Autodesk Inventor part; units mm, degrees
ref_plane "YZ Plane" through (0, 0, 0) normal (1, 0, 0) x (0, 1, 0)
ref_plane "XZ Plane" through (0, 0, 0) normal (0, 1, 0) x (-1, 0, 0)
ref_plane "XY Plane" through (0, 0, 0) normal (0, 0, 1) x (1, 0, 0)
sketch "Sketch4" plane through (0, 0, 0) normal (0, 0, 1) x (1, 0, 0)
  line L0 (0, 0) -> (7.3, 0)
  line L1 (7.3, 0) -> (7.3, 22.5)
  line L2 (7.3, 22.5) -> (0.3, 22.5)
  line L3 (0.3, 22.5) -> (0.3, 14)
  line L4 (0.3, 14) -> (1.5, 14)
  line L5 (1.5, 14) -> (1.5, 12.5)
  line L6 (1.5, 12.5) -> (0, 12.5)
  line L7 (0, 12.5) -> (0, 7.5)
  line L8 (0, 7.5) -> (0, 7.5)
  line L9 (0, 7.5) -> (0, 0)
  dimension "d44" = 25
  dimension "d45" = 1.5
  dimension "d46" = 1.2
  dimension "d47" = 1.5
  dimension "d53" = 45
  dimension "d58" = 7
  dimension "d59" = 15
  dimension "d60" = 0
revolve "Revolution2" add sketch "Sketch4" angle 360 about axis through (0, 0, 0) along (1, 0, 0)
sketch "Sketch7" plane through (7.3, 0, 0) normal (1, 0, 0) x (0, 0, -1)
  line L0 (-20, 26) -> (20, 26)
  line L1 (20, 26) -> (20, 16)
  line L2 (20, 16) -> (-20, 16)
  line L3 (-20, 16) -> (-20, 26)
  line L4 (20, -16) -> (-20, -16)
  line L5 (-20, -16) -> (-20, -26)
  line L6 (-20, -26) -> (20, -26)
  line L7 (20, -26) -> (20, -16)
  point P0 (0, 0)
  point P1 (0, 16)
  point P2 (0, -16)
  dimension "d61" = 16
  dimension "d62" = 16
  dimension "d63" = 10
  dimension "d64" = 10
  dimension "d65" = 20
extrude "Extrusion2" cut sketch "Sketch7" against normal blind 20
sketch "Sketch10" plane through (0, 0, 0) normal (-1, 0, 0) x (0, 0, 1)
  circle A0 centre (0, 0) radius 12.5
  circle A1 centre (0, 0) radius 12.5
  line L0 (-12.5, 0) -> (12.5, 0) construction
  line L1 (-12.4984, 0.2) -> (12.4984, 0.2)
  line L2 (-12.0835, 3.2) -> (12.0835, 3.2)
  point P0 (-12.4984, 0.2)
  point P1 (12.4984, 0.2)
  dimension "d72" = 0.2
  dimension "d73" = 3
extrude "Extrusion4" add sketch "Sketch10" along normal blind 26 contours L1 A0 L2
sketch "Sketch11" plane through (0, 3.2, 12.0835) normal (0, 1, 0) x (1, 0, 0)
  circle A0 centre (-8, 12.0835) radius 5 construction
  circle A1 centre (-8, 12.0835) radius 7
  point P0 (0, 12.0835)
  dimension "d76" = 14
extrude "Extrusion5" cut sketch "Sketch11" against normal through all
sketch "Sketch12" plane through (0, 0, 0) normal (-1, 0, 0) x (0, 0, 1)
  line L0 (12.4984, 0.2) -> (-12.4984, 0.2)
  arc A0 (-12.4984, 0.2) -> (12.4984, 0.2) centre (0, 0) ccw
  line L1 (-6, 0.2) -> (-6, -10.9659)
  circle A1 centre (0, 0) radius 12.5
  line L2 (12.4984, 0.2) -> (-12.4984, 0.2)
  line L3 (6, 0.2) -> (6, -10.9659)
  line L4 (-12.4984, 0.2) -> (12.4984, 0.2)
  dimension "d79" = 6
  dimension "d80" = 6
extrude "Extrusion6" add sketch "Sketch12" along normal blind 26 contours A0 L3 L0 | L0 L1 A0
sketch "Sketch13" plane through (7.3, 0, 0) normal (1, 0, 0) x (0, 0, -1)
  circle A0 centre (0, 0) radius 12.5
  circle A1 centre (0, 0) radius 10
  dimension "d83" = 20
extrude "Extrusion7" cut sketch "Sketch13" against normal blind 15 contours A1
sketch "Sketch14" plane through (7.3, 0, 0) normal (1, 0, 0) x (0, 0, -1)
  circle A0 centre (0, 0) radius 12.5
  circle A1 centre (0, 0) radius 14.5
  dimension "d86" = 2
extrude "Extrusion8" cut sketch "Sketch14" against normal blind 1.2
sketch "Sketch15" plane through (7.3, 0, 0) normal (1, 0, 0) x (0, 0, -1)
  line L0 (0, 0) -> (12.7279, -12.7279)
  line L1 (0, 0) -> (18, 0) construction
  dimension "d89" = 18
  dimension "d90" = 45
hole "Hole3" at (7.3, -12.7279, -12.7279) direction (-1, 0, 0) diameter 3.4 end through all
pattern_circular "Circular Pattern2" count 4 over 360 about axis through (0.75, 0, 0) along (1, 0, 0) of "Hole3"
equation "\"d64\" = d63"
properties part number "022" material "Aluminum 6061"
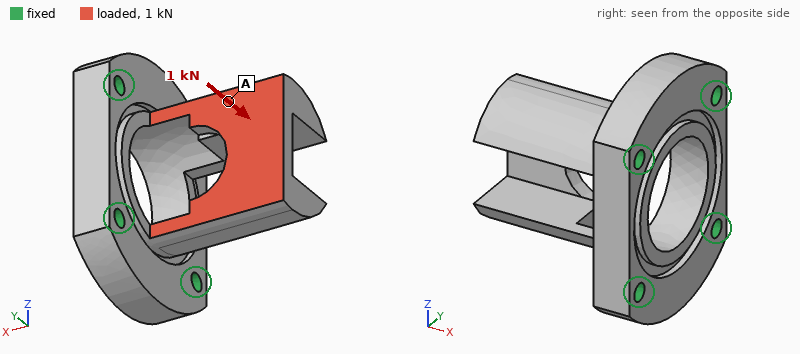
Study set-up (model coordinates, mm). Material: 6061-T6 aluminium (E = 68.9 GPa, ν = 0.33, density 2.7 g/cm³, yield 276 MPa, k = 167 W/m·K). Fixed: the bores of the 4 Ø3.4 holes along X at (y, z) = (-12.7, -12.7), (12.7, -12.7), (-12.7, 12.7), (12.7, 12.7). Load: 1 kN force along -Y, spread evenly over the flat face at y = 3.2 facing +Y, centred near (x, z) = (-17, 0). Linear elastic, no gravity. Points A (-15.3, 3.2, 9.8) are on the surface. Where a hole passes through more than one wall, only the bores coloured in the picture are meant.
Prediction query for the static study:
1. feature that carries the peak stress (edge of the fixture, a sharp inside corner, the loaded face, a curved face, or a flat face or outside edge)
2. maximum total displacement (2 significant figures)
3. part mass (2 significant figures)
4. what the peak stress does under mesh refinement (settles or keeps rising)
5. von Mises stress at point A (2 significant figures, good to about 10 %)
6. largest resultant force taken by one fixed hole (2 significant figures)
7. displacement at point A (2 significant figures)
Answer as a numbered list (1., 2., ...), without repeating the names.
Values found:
1. a sharp inside corner
2. 0.12 mm
3. 27 g
4. keeps rising
5. 18 MPa
6. 580 N
7. 0.061 mm
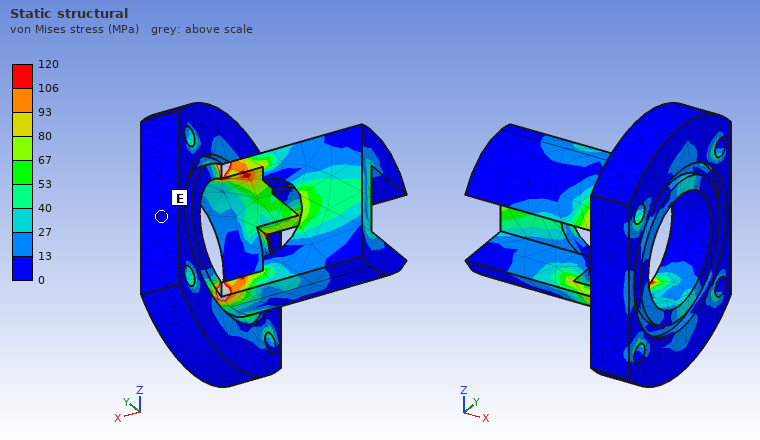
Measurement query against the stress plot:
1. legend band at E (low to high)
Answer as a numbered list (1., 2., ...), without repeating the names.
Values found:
1. 0 to 13 MPa
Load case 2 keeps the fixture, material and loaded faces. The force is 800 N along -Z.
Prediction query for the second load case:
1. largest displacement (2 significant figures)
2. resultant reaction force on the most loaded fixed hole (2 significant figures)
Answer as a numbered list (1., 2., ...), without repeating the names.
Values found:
1. 81 µm
2. 500 N
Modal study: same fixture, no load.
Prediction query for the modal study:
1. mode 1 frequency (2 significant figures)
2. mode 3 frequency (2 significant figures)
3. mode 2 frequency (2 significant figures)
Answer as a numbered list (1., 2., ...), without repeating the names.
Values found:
1. 6200 Hz
2. 10 kHz
3. 6300 Hz
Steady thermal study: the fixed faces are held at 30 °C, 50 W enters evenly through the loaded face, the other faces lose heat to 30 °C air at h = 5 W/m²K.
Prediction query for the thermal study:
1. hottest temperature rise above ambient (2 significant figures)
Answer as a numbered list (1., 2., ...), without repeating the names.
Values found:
1. 77 K
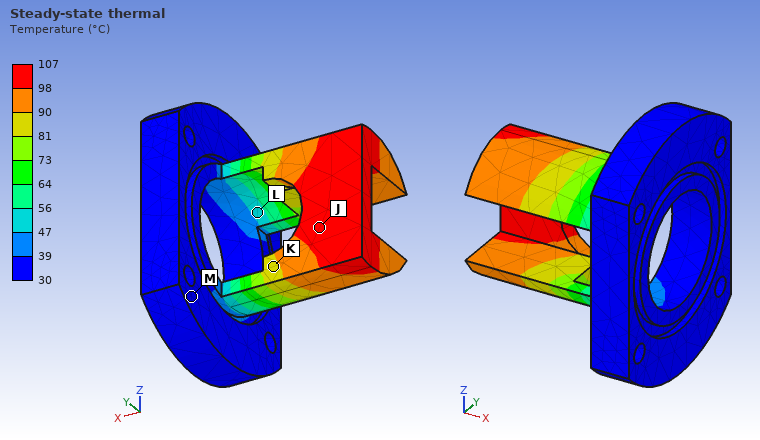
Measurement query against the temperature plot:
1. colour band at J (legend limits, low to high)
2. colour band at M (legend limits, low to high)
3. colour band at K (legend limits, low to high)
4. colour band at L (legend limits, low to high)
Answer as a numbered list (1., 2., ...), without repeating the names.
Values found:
1. 98 to 107 °C
2. 30 to 39 °C
3. 81 to 90 °C
4. 47 to 56 °C
